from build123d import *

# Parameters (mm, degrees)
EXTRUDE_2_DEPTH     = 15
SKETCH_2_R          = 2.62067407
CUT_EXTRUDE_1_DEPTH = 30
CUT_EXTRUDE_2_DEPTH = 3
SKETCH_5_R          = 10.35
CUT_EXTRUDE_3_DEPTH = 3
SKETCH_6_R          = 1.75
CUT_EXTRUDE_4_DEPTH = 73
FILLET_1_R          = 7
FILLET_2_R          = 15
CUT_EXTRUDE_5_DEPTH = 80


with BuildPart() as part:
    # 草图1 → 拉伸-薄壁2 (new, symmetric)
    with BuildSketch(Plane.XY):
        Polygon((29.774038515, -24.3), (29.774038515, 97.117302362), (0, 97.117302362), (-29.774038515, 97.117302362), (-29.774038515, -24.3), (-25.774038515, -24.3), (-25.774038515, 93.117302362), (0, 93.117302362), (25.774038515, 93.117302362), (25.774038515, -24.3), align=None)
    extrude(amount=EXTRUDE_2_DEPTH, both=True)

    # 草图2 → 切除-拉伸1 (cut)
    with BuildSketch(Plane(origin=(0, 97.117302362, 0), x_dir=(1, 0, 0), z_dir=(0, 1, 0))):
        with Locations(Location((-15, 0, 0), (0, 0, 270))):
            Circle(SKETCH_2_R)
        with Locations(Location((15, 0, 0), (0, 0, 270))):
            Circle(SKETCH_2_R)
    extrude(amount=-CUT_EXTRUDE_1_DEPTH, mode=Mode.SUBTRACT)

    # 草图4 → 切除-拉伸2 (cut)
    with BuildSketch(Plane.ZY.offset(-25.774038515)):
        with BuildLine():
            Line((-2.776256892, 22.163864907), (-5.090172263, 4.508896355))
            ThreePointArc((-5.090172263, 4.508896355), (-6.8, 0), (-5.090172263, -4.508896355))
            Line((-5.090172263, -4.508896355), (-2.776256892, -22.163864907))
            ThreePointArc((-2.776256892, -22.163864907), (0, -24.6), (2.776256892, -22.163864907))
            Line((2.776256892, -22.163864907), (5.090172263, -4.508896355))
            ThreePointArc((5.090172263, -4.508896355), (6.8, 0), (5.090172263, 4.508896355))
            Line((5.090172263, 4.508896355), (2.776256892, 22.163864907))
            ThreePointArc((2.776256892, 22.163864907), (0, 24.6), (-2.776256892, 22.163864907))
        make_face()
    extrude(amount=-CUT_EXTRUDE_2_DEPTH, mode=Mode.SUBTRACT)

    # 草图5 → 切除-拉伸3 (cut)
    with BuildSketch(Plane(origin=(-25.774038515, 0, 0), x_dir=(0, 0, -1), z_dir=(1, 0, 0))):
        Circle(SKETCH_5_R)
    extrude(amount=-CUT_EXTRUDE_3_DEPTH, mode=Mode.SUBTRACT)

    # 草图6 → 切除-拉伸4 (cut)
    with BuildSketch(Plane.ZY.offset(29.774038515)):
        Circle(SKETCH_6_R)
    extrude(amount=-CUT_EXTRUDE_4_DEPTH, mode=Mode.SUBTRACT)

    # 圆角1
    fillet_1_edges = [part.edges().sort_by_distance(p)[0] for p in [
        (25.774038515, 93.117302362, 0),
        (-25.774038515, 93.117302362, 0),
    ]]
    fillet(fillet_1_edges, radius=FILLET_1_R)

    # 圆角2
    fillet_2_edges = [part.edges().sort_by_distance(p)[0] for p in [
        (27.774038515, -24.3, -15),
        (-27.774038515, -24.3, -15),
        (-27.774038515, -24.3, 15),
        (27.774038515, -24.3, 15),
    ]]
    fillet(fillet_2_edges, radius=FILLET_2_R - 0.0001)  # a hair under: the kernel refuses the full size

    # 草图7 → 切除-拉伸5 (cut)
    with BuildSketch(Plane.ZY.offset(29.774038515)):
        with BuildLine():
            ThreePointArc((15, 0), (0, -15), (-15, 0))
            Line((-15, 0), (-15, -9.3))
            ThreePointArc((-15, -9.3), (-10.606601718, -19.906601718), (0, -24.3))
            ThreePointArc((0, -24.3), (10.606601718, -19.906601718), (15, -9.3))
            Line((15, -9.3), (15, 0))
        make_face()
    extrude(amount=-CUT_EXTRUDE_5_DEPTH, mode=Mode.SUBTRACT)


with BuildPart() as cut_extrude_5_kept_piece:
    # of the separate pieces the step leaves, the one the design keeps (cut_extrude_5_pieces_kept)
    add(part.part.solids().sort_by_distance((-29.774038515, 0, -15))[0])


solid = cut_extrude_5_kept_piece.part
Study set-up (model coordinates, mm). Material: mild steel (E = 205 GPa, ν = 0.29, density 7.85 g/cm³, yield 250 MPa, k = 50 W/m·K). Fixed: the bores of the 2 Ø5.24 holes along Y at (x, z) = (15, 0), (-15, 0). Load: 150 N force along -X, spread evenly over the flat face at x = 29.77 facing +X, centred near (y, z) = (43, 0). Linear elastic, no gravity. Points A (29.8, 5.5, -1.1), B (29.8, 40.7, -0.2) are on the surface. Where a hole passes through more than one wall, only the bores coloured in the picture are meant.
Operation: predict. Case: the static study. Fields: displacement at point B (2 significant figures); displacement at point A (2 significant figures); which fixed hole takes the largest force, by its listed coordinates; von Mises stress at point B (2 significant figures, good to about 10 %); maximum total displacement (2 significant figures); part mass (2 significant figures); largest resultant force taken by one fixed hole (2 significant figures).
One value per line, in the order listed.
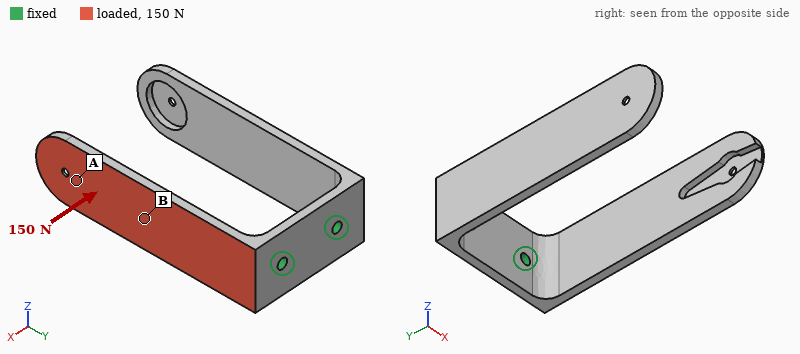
0.30 mm
0.61 mm
(15, 0)
24 MPa
0.81 mm
240 g
160 N
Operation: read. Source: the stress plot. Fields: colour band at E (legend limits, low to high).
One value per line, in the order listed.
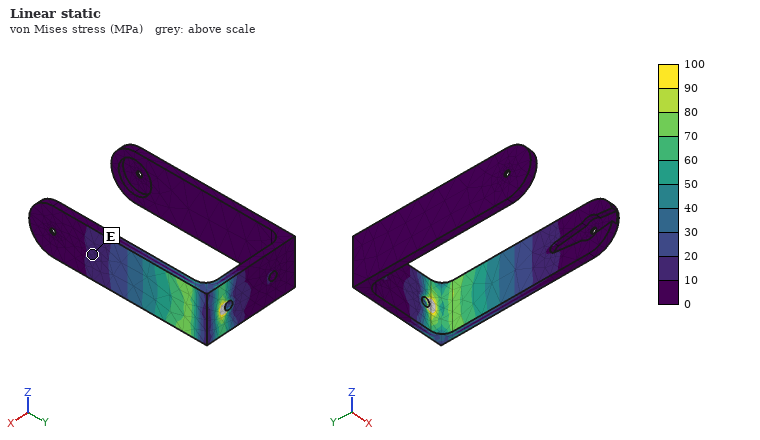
10 to 20 MPa
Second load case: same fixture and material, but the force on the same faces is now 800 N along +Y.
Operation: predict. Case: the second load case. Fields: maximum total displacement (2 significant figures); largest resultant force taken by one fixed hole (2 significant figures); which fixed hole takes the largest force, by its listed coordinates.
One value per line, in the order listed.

0.40 mm
880 N
(15, 0)
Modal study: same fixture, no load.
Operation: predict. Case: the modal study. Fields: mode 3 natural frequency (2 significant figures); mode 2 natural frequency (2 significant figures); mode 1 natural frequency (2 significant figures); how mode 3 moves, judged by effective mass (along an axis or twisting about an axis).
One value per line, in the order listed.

700 Hz
310 Hz
310 Hz
along Z
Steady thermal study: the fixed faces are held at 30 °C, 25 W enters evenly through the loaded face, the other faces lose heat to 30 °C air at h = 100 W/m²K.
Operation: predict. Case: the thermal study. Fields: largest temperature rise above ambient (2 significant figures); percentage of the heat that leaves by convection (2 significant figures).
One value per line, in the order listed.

48 K
73 %
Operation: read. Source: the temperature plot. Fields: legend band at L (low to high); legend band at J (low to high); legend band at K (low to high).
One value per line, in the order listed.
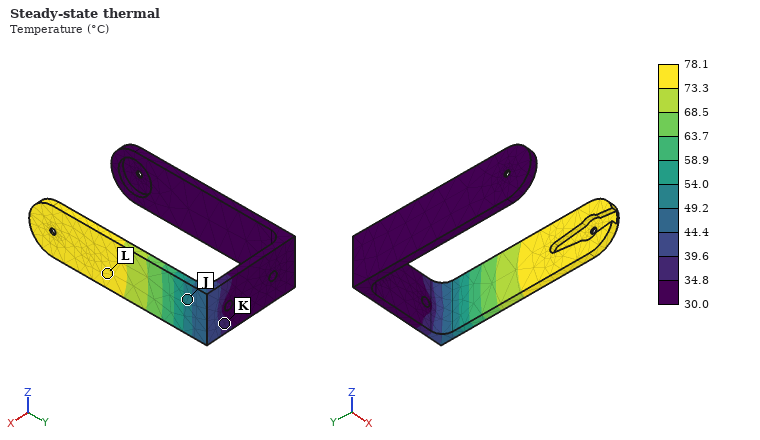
73.3 to 78.1 °C
49.2 to 54.0 °C
34.8 to 39.6 °C
